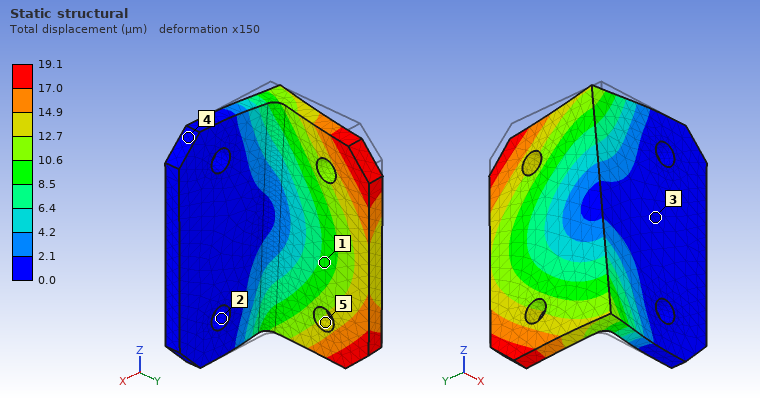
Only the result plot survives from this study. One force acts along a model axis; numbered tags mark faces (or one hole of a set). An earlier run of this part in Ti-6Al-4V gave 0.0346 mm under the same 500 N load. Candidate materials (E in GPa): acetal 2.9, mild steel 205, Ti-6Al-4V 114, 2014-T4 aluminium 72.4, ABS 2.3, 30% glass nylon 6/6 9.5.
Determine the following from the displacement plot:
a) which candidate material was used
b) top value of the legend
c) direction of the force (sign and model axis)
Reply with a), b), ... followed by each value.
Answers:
a) mild steel
b) 19.1 µm
c) -Z
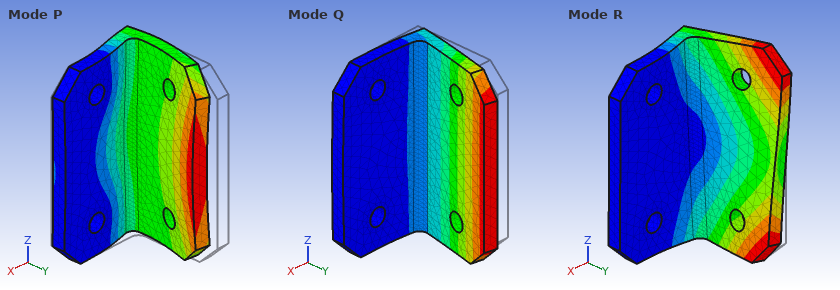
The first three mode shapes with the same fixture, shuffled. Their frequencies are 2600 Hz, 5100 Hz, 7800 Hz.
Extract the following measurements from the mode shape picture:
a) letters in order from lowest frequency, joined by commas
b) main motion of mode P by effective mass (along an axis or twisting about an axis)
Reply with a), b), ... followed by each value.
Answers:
a) Q, R, P
b) along Y
